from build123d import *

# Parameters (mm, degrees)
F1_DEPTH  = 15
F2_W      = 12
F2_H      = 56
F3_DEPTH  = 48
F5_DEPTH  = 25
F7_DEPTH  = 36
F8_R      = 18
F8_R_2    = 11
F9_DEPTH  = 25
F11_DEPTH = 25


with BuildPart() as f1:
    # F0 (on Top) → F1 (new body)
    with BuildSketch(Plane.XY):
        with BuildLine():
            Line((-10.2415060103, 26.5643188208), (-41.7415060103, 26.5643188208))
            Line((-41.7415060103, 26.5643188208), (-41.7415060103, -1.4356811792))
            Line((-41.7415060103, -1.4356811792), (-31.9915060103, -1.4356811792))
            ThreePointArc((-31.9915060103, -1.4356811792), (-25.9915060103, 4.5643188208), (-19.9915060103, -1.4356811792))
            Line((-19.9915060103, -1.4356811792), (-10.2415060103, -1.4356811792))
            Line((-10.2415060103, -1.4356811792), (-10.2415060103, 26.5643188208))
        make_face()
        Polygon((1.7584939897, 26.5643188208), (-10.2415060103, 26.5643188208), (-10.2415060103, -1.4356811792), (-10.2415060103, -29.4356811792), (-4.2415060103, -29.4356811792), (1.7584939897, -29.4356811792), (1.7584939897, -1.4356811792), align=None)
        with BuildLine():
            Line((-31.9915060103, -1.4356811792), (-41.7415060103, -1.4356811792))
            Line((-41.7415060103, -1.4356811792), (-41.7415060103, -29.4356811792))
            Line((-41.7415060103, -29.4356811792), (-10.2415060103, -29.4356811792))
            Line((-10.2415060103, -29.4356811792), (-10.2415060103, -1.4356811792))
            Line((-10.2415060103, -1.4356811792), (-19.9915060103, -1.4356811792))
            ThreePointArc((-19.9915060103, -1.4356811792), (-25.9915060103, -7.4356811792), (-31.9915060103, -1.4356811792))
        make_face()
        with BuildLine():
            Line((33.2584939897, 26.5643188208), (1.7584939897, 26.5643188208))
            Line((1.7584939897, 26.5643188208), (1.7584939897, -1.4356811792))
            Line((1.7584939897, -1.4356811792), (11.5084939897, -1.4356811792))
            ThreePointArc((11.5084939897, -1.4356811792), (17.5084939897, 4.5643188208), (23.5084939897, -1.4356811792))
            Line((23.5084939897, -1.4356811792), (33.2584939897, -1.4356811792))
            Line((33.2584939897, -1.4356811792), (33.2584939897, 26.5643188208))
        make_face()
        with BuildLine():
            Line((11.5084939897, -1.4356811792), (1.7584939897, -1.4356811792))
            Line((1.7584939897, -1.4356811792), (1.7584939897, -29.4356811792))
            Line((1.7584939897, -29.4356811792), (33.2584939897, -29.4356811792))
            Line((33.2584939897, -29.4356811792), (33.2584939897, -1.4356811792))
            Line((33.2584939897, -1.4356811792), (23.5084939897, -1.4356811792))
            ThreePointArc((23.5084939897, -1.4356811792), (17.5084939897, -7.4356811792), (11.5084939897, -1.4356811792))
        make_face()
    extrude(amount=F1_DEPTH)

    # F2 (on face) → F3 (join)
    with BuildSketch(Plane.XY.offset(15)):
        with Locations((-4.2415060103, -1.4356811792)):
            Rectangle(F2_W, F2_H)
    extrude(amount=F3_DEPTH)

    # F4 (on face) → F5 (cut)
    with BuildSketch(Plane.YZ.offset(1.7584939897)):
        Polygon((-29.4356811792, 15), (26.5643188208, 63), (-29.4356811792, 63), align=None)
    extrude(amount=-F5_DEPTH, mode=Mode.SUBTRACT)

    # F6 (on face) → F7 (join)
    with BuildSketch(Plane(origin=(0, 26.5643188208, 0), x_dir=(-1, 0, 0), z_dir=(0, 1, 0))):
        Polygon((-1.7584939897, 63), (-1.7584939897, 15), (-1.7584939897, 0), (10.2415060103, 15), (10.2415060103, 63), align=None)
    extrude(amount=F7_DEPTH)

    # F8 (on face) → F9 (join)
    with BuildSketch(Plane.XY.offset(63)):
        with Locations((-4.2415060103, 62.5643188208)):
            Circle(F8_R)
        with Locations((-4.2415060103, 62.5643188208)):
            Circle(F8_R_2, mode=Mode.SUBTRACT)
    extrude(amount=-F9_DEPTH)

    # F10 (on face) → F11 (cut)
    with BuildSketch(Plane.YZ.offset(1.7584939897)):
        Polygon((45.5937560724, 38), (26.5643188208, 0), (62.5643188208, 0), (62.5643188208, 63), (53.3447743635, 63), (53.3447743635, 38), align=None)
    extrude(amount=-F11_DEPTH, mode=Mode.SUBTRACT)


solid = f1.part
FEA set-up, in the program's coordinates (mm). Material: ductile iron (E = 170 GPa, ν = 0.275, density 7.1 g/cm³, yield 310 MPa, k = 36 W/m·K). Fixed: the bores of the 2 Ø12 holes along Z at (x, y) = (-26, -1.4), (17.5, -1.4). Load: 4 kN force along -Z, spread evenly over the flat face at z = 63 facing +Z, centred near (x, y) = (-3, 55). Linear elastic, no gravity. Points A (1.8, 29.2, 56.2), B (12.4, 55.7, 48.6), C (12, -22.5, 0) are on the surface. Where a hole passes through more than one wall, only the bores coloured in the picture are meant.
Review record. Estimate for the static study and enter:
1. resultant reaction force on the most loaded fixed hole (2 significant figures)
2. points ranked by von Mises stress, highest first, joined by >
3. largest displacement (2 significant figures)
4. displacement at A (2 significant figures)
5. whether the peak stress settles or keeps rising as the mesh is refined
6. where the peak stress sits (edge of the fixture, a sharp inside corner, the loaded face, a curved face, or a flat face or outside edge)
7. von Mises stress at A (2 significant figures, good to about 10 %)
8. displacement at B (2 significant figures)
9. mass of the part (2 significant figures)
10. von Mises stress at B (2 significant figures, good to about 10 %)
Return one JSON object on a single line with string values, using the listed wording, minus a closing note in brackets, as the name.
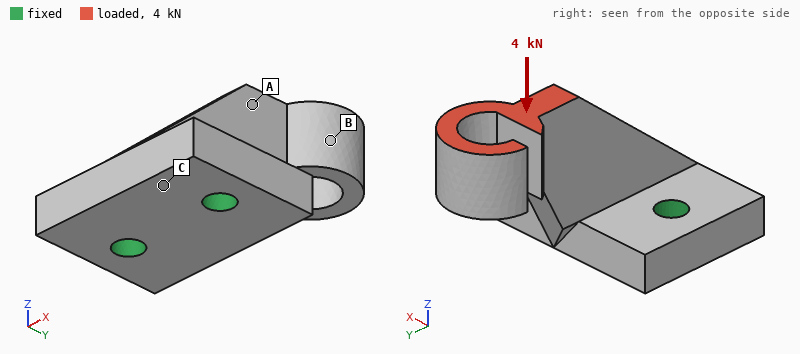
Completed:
{"resultant reaction force on the most loaded fixed hole": "2.4 kN", "points ranked by von Mises stress, highest first, joined by >": "B > A > C", "largest displacement": "0.22 mm", "displacement at A": "0.050 mm", "whether the peak stress settles or keeps rising as the mesh is refined": "keeps rising", "where the peak stress sits": "a sharp inside corner", "von Mises stress at A": "30 MPa", "displacement at B": "0.069 mm", "mass of the part": "710 g", "von Mises stress at B": "92 MPa"}
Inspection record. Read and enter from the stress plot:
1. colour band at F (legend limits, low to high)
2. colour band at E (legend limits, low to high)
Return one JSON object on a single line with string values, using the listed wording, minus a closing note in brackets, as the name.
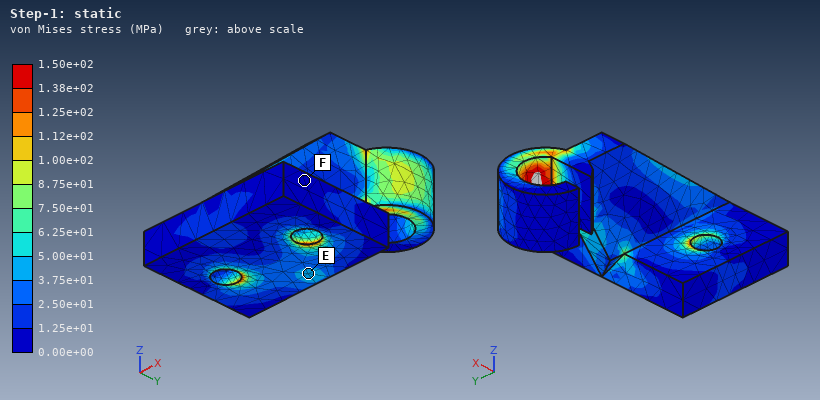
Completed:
{"colour band at F": "0.00e+00 to 1.25e+01 MPa", "colour band at E": "3.75e+01 to 5.00e+01 MPa"}
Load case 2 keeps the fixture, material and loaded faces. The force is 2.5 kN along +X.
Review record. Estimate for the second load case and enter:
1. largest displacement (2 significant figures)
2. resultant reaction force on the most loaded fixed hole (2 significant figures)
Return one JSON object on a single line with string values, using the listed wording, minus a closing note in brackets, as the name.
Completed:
{"largest displacement": "0.48 mm", "resultant reaction force on the most loaded fixed hole": "4.9 kN"}
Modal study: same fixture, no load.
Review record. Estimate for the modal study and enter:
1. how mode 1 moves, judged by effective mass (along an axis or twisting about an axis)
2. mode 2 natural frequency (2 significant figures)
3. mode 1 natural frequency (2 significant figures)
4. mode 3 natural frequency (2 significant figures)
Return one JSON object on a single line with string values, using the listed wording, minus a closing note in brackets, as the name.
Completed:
{"how mode 1 moves, judged by effective mass": "along X", "mode 2 natural frequency": "2000 Hz", "mode 1 natural frequency": "1300 Hz", "mode 3 natural frequency": "2500 Hz"}
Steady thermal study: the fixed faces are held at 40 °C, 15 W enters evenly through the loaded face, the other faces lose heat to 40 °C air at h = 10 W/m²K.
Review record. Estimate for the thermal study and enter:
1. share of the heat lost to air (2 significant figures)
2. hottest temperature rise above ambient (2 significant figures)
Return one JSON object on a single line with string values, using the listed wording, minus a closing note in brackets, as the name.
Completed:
{"share of the heat lost to air": "27 %", "hottest temperature rise above ambient": "77 K"}
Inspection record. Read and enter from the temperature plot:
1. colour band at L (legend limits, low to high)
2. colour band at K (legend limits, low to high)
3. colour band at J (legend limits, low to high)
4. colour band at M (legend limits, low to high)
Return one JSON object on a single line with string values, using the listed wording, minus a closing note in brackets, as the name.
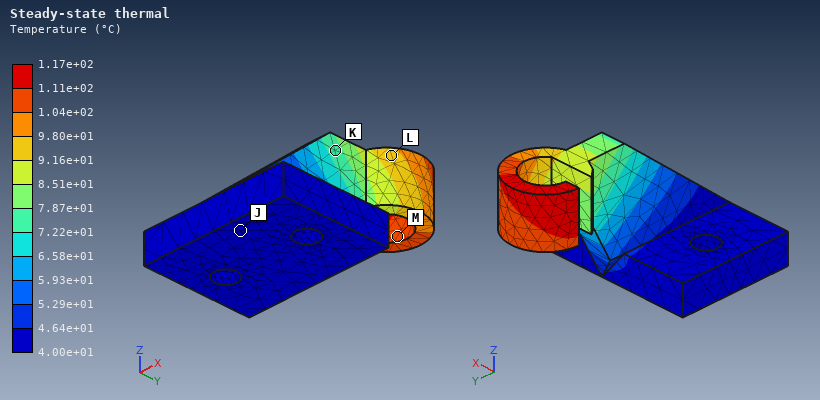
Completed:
{"colour band at L": "9.16e+01 to 9.80e+01 °C", "colour band at K": "7.22e+01 to 7.87e+01 °C", "colour band at J": "4.00e+01 to 4.64e+01 °C", "colour band at M": "1.04e+02 to 1.11e+02 °C"}
